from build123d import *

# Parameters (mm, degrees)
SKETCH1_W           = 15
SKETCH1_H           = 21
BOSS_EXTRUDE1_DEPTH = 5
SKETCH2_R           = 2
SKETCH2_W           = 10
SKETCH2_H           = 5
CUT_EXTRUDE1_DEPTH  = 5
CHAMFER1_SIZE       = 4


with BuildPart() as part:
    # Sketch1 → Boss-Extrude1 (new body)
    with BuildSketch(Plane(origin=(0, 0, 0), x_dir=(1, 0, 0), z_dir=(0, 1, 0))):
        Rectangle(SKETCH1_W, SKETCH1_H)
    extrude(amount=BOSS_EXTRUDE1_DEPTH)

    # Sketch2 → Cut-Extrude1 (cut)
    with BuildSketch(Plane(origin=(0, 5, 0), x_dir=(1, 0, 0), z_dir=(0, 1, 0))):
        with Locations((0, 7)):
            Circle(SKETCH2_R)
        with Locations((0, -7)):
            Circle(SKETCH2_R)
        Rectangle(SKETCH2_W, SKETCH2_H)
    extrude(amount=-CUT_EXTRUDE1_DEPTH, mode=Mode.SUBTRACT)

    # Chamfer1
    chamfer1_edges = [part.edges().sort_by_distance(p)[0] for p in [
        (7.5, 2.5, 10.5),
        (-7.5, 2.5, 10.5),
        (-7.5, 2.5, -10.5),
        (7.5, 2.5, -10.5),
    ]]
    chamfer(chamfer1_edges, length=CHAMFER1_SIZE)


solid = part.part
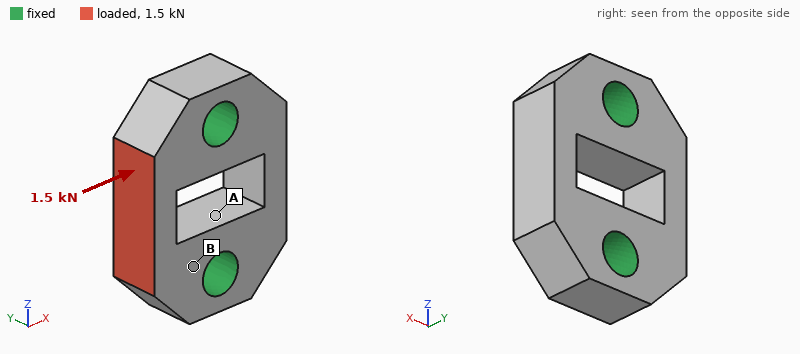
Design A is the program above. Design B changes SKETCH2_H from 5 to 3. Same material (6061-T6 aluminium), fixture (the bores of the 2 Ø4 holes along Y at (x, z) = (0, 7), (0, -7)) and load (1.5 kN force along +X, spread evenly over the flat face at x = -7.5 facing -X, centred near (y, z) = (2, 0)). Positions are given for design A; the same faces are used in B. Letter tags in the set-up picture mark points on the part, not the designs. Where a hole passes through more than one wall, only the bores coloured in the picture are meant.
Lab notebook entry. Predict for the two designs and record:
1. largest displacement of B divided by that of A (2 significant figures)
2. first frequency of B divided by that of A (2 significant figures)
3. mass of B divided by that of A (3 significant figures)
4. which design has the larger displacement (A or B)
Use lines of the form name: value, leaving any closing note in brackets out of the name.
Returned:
largest displacement of B divided by that of A: 0.63
first frequency of B divided by that of A: 1.00
mass of B divided by that of A: 1.10
which design has the larger displacement: A
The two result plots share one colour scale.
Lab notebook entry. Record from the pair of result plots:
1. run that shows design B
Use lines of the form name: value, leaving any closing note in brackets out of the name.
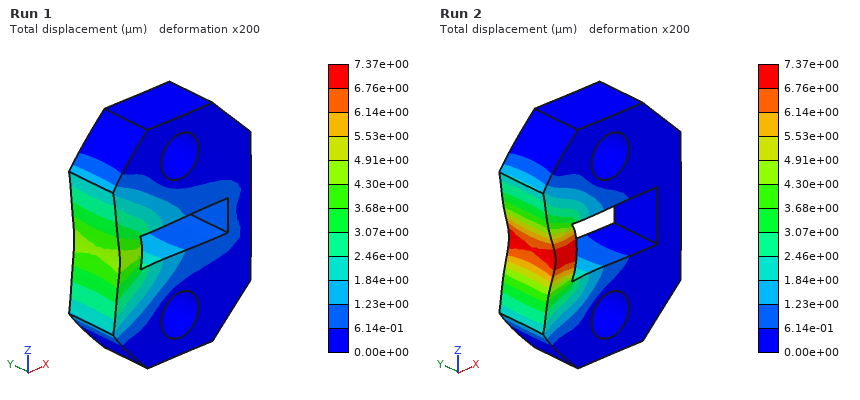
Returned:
run that shows design B: Run 1
